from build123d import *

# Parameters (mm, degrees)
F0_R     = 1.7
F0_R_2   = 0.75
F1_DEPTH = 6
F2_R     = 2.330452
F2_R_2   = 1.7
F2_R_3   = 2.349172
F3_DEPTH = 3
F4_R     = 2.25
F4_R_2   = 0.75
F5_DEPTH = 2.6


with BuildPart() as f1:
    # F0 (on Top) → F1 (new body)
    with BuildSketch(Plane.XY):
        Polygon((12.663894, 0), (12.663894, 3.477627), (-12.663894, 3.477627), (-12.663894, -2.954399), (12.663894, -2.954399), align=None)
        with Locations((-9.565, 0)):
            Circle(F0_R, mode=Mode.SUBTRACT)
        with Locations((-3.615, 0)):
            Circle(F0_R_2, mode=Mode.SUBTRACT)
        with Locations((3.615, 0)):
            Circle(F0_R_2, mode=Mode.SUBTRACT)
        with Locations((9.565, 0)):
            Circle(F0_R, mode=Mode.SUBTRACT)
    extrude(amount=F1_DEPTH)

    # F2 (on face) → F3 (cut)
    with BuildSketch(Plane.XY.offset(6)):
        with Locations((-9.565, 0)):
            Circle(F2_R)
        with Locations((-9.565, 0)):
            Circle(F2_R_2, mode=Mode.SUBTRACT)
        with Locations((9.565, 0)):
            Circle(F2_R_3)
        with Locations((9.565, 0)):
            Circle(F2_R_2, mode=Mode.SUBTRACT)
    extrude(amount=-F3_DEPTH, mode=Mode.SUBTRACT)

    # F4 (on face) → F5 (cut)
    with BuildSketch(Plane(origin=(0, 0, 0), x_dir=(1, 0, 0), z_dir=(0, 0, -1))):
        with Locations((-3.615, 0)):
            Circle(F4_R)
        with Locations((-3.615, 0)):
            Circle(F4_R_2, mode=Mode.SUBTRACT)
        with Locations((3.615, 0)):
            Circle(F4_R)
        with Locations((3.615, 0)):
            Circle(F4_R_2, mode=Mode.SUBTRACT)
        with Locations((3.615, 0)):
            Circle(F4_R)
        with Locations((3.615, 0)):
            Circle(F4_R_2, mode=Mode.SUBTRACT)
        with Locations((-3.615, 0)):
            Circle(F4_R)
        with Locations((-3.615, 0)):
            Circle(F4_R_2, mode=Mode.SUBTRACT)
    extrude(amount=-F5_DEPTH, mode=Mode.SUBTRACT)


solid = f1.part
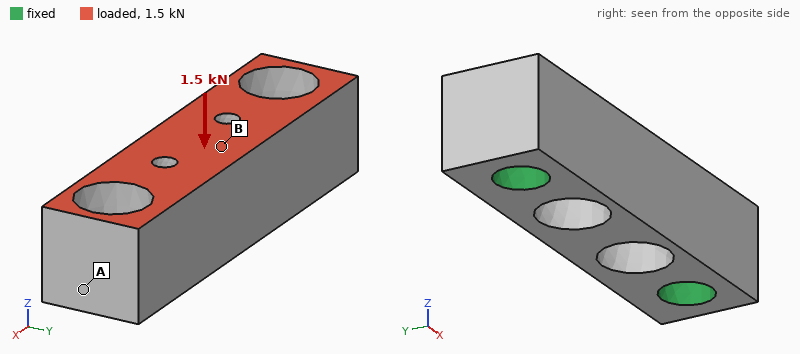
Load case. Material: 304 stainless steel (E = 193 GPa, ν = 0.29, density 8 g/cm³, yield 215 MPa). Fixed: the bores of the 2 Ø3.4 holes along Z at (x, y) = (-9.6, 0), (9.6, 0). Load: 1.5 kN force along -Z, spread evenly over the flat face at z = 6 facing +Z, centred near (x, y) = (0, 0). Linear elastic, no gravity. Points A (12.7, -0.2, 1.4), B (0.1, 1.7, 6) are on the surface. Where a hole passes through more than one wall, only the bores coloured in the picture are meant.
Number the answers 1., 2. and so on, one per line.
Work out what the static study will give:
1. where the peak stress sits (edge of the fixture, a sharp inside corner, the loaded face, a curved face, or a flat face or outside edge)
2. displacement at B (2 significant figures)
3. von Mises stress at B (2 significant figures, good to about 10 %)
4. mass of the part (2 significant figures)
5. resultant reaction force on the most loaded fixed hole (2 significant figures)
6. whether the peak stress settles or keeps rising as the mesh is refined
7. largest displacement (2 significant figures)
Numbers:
1. edge of the fixture
2. 3.4 µm
3. 43 MPa
4. 5.8 g
5. 810 N
6. keeps rising
7. 3.5 µm
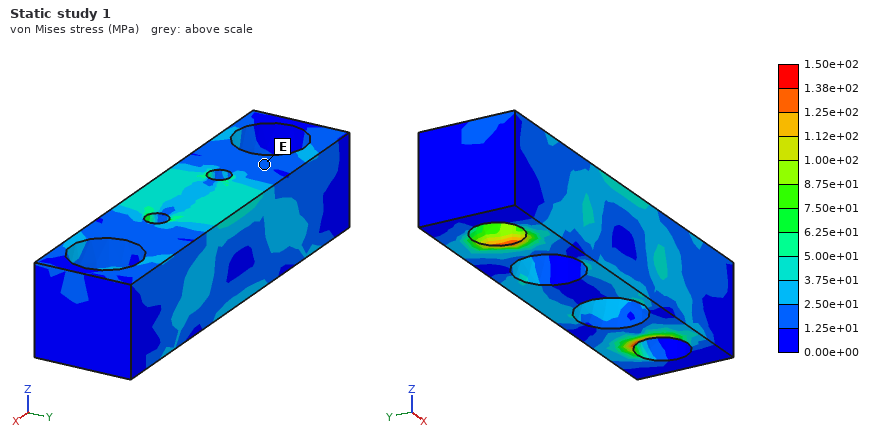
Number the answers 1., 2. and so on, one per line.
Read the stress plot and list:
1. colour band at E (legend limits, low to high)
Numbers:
1. 1.25e+01 to 2.50e+01 MPa
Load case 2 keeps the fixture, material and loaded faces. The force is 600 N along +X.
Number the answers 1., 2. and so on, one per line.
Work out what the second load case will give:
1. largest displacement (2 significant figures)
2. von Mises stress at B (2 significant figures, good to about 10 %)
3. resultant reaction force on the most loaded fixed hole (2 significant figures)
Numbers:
1. 1.1 µm
2. 8.5 MPa
3. 320 N
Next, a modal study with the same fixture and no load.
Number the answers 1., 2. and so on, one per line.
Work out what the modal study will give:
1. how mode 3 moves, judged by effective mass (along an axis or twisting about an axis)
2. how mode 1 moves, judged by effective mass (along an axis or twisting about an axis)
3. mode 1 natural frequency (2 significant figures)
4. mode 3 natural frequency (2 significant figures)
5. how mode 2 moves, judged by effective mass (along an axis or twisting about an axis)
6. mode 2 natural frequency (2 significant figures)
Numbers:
1. twisting about X
2. along Y
3. 45 kHz
4. 56 kHz
5. along Z
6. 51 kHz
